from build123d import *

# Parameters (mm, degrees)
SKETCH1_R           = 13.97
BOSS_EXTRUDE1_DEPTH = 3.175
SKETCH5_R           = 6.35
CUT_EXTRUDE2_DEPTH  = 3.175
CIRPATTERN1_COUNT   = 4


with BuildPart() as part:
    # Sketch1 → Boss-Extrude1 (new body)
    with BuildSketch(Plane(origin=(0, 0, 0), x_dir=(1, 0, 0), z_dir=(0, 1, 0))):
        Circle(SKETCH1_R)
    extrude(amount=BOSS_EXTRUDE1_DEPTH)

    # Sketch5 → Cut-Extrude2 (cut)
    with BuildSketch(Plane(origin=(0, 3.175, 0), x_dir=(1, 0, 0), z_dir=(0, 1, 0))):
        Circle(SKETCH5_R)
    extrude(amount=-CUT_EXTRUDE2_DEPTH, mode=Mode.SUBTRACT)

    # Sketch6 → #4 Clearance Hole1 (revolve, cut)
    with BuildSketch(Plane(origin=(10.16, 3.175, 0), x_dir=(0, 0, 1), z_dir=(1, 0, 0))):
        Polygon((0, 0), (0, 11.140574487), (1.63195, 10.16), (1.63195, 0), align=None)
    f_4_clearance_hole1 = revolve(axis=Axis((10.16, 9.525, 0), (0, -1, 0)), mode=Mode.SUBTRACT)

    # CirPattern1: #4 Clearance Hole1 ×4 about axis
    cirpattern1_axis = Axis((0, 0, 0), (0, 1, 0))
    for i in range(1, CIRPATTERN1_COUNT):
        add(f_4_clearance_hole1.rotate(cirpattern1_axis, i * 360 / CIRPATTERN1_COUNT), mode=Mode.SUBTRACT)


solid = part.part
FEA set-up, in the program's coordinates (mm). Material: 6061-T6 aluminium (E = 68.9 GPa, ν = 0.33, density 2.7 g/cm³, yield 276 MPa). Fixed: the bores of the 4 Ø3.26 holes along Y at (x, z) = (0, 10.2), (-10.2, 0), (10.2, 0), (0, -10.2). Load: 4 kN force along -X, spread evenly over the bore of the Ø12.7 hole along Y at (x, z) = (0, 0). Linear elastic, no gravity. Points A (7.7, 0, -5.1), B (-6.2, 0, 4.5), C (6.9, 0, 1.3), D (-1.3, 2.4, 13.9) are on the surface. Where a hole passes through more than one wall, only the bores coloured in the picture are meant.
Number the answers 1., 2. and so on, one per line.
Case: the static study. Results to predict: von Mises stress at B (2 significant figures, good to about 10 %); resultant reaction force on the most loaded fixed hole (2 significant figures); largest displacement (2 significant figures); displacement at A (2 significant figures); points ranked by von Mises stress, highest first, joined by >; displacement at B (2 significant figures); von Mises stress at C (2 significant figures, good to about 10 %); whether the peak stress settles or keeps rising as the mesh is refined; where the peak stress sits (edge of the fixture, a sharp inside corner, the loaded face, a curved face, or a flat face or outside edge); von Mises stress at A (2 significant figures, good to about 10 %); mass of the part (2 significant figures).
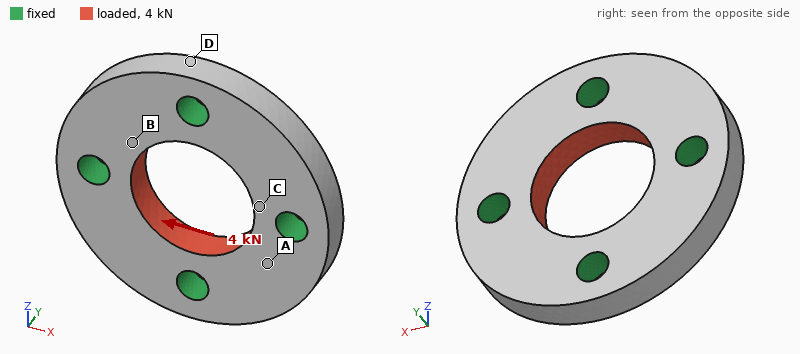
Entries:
1. 33 MPa
2. 1.0 kN
3. 4.4 µm
4. 3.1 µm
5. C > B > A > D
6. 3.6 µm
7. 48 MPa
8. keeps rising
9. edge of the fixture
10. 23 MPa
11. 3.9 g
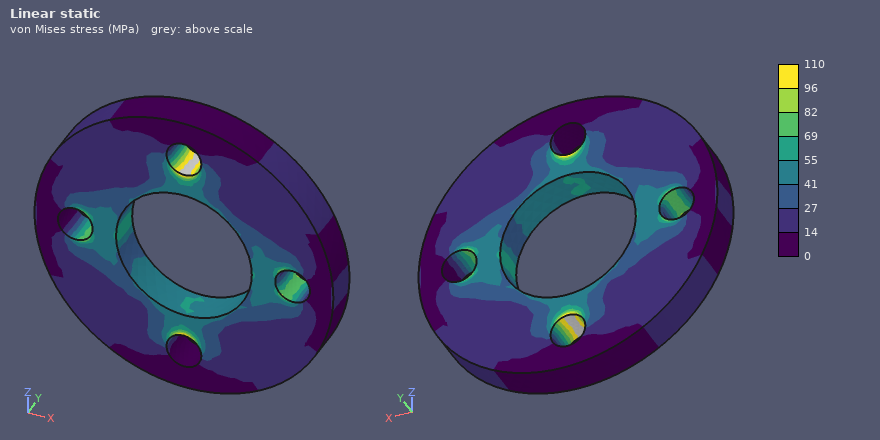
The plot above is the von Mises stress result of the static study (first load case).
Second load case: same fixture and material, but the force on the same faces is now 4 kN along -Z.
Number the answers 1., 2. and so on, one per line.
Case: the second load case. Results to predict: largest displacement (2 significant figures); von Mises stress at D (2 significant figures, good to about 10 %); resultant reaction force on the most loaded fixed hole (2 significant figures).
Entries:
1. 4.4 µm
2. 14 MPa
3. 1.0 kN
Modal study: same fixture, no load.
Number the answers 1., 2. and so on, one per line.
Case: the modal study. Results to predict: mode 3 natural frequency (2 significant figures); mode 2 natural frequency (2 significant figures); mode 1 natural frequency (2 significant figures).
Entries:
1. 51 kHz
2. 51 kHz
3. 50 kHz
